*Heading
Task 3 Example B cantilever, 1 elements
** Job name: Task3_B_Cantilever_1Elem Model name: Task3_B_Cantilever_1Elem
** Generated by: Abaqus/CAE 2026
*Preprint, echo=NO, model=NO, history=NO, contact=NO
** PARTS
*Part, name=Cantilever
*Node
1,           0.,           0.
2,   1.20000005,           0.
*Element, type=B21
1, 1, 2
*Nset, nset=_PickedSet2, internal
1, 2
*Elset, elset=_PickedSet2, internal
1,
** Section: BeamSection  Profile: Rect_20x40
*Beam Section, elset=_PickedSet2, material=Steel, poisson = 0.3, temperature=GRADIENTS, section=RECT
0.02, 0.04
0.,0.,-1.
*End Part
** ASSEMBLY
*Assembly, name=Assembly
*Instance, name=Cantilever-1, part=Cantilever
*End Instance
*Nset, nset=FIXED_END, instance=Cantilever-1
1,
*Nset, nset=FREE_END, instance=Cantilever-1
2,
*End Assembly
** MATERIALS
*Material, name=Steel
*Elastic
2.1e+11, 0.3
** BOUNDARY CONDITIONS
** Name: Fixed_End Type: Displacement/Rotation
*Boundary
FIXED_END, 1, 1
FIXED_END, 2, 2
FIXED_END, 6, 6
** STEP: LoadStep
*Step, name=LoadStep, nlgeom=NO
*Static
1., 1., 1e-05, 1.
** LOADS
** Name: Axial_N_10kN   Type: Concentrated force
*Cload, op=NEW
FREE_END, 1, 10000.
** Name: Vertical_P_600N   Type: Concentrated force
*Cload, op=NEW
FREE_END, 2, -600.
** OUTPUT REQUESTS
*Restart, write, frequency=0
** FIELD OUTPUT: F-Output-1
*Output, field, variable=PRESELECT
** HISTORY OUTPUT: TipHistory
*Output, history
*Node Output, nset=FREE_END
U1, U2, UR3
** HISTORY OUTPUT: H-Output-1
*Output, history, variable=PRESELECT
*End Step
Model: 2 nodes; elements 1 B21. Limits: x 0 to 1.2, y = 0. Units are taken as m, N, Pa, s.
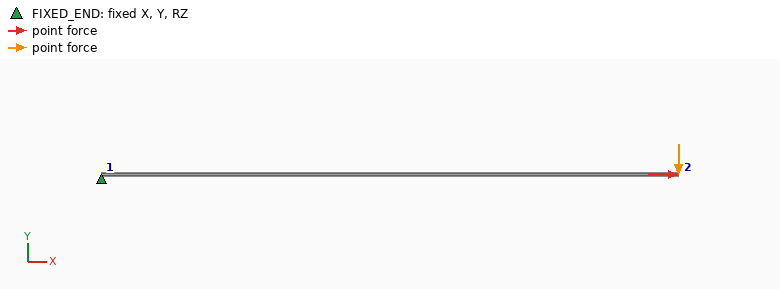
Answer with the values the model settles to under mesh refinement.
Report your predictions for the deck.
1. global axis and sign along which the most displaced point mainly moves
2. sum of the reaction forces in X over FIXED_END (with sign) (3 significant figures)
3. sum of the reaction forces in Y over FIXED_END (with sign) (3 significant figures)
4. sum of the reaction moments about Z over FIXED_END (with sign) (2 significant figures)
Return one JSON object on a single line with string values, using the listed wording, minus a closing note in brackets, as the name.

{"global axis and sign along which the most displaced point mainly moves": "-Y", "sum of the reaction forces in X over FIXED_END (with sign)": "-10000 N", "sum of the reaction forces in Y over FIXED_END (with sign)": "600 N", "sum of the reaction moments about Z over FIXED_END (with sign)": "720 N·m"}
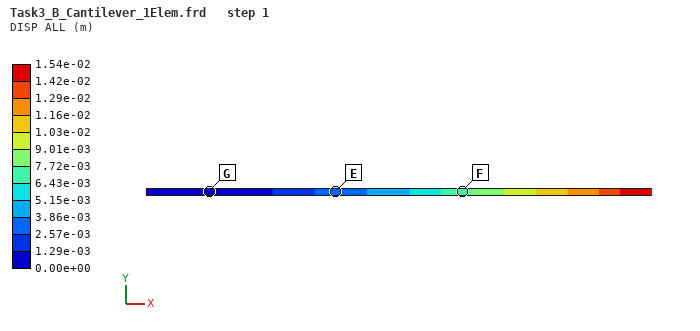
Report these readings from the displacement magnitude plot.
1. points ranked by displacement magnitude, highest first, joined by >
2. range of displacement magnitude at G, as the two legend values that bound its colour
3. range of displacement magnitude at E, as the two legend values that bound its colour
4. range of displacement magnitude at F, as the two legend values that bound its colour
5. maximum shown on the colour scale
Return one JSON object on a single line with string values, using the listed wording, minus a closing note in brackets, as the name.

{"points ranked by displacement magnitude, highest first, joined by >": "F > E > G", "range of displacement magnitude at G, as the two legend values that bound its colour": "0.00e+00 to 1.29e-03 m", "range of displacement magnitude at E, as the two legend values that bound its colour": "2.57e-03 to 3.86e-03 m", "range of displacement magnitude at F, as the two legend values that bound its colour": "6.43e-03 to 7.72e-03 m", "maximum shown on the colour scale": "1.54e-02 m"}
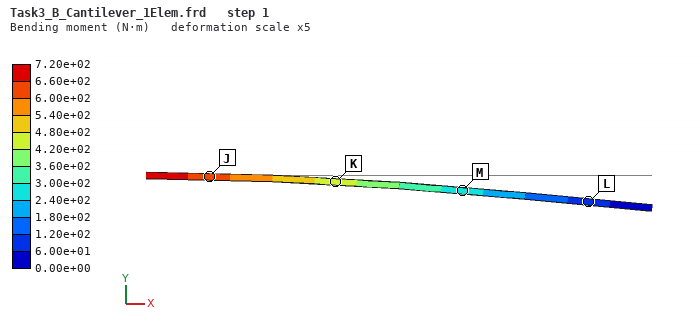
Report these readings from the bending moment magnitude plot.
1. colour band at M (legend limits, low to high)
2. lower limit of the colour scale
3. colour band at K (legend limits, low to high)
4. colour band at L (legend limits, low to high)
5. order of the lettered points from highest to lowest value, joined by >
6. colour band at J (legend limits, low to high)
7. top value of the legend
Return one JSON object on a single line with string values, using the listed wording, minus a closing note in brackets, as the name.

{"colour band at M": "2.40e+02 to 3.00e+02 N·m", "lower limit of the colour scale": "0.00e+00 N·m", "colour band at K": "4.20e+02 to 4.80e+02 N·m", "colour band at L": "6.00e+01 to 1.20e+02 N·m", "order of the lettered points from highest to lowest value, joined by >": "J > K > M > L", "colour band at J": "6.00e+02 to 6.60e+02 N·m", "top value of the legend": "7.20e+02 N·m"}
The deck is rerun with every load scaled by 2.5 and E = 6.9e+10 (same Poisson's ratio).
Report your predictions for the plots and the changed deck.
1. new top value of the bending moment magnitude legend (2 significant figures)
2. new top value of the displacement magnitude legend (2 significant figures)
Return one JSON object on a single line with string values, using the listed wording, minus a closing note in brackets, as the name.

{"new top value of the bending moment magnitude legend": "1800 N·m", "new top value of the displacement magnitude legend": "0.12 m"}
